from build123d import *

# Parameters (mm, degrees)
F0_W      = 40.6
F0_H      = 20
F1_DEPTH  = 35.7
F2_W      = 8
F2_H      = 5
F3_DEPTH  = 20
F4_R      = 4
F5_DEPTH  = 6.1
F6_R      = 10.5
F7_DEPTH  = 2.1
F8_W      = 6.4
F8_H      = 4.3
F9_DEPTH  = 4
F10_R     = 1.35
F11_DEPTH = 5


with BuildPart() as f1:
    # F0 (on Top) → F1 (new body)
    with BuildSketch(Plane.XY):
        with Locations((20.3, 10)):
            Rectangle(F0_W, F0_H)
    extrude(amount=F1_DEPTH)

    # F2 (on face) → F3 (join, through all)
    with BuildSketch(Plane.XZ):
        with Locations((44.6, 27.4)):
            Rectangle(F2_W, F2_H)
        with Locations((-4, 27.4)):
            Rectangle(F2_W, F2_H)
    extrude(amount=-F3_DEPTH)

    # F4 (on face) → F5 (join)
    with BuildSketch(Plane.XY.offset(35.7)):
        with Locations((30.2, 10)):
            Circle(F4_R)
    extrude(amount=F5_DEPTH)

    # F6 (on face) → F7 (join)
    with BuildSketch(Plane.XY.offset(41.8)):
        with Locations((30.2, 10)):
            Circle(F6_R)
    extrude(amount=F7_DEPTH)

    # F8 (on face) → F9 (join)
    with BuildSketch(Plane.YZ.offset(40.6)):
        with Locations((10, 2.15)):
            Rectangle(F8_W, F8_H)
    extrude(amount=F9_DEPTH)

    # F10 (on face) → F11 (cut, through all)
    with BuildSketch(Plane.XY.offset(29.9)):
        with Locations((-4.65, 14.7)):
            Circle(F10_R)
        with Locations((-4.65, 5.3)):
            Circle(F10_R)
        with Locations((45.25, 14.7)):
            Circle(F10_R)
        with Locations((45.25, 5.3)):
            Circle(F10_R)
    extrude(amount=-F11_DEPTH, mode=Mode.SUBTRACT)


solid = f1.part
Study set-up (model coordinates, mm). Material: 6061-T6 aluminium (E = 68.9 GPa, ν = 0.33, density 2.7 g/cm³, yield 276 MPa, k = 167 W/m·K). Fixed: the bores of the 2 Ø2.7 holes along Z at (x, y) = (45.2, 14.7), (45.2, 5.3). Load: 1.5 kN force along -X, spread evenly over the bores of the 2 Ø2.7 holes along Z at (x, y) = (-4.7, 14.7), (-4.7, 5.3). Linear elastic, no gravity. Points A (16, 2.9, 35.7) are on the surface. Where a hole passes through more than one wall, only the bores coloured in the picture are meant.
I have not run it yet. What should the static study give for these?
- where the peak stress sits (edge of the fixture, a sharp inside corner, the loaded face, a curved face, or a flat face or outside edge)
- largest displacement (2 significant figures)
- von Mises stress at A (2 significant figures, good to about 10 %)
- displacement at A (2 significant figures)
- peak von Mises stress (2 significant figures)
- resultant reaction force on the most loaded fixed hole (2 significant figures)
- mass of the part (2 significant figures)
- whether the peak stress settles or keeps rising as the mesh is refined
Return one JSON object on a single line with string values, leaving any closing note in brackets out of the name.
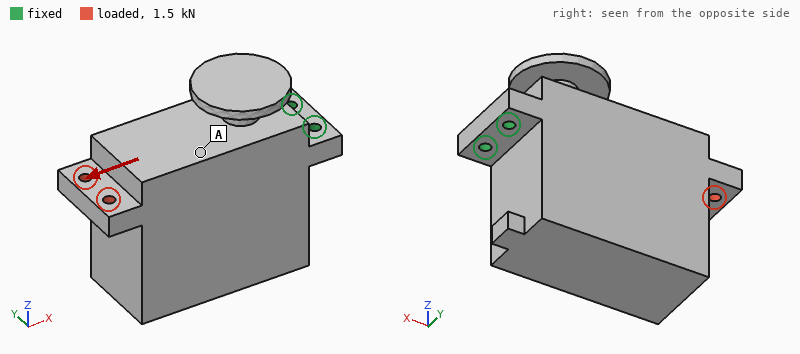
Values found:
{"where the peak stress sits": "the loaded face", "largest displacement": "7.5 µm", "von Mises stress at A": "5.2 MPa", "displacement at A": "3.6 µm", "peak von Mises stress": "47 MPa", "resultant reaction force on the most loaded fixed hole": "750 N", "mass of the part": "85 g", "whether the peak stress settles or keeps rising as the mesh is refined": "settles"}
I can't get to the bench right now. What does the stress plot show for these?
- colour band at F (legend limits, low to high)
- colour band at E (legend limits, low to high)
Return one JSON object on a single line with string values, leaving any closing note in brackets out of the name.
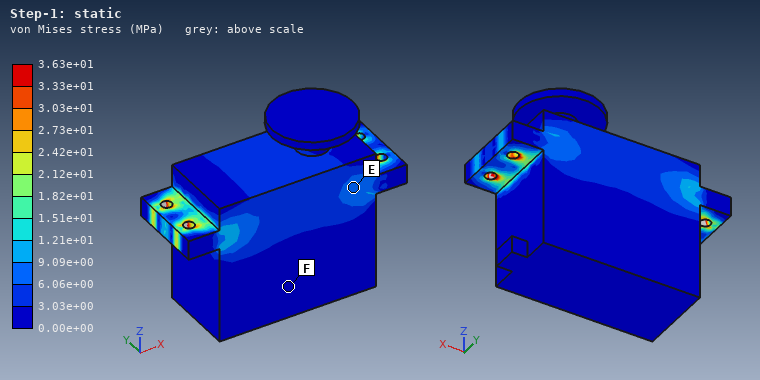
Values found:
{"colour band at F": "0.00e+00 to 3.03e+00 MPa", "colour band at E": "6.06e+00 to 9.09e+00 MPa"}
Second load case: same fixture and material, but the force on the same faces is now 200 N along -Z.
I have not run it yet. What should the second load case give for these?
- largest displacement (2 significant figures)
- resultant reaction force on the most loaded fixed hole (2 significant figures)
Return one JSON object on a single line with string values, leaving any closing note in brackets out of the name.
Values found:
{"largest displacement": "0.21 mm", "resultant reaction force on the most loaded fixed hole": "100 N"}
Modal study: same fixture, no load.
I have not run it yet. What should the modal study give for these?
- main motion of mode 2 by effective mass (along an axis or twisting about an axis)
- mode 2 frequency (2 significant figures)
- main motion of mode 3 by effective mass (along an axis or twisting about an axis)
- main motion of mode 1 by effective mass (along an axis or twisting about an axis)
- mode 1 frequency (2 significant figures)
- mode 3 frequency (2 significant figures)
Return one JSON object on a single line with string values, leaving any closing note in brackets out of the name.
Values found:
{"main motion of mode 2 by effective mass": "along Y", "mode 2 frequency": "2400 Hz", "main motion of mode 3 by effective mass": "twisting about X", "main motion of mode 1 by effective mass": "along Z", "mode 1 frequency": "900 Hz", "mode 3 frequency": "4200 Hz"}
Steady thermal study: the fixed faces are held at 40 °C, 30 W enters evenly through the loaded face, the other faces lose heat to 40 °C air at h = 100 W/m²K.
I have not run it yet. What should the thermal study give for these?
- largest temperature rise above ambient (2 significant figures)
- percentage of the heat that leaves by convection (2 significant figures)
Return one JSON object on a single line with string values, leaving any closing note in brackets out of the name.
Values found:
{"largest temperature rise above ambient": "34 K", "percentage of the heat that leaves by convection": "33 %"}
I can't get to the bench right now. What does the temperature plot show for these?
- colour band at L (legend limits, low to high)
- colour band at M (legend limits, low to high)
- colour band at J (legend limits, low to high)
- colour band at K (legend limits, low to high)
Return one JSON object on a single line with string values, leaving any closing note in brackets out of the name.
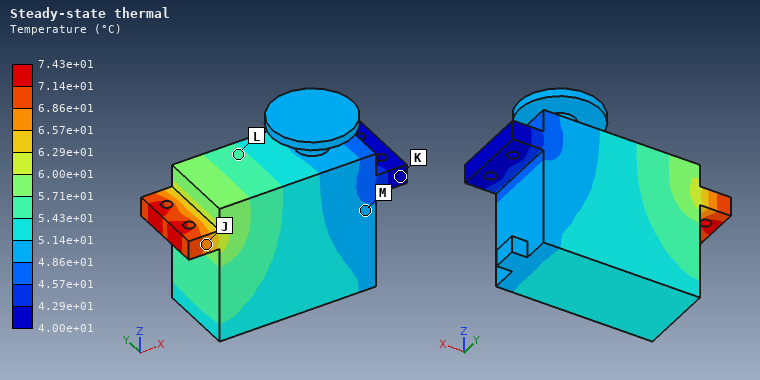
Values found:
{"colour band at L": "5.43e+01 to 5.71e+01 °C", "colour band at M": "4.86e+01 to 5.14e+01 °C", "colour band at J": "6.57e+01 to 6.86e+01 °C", "colour band at K": "4.00e+01 to 4.29e+01 °C"}
